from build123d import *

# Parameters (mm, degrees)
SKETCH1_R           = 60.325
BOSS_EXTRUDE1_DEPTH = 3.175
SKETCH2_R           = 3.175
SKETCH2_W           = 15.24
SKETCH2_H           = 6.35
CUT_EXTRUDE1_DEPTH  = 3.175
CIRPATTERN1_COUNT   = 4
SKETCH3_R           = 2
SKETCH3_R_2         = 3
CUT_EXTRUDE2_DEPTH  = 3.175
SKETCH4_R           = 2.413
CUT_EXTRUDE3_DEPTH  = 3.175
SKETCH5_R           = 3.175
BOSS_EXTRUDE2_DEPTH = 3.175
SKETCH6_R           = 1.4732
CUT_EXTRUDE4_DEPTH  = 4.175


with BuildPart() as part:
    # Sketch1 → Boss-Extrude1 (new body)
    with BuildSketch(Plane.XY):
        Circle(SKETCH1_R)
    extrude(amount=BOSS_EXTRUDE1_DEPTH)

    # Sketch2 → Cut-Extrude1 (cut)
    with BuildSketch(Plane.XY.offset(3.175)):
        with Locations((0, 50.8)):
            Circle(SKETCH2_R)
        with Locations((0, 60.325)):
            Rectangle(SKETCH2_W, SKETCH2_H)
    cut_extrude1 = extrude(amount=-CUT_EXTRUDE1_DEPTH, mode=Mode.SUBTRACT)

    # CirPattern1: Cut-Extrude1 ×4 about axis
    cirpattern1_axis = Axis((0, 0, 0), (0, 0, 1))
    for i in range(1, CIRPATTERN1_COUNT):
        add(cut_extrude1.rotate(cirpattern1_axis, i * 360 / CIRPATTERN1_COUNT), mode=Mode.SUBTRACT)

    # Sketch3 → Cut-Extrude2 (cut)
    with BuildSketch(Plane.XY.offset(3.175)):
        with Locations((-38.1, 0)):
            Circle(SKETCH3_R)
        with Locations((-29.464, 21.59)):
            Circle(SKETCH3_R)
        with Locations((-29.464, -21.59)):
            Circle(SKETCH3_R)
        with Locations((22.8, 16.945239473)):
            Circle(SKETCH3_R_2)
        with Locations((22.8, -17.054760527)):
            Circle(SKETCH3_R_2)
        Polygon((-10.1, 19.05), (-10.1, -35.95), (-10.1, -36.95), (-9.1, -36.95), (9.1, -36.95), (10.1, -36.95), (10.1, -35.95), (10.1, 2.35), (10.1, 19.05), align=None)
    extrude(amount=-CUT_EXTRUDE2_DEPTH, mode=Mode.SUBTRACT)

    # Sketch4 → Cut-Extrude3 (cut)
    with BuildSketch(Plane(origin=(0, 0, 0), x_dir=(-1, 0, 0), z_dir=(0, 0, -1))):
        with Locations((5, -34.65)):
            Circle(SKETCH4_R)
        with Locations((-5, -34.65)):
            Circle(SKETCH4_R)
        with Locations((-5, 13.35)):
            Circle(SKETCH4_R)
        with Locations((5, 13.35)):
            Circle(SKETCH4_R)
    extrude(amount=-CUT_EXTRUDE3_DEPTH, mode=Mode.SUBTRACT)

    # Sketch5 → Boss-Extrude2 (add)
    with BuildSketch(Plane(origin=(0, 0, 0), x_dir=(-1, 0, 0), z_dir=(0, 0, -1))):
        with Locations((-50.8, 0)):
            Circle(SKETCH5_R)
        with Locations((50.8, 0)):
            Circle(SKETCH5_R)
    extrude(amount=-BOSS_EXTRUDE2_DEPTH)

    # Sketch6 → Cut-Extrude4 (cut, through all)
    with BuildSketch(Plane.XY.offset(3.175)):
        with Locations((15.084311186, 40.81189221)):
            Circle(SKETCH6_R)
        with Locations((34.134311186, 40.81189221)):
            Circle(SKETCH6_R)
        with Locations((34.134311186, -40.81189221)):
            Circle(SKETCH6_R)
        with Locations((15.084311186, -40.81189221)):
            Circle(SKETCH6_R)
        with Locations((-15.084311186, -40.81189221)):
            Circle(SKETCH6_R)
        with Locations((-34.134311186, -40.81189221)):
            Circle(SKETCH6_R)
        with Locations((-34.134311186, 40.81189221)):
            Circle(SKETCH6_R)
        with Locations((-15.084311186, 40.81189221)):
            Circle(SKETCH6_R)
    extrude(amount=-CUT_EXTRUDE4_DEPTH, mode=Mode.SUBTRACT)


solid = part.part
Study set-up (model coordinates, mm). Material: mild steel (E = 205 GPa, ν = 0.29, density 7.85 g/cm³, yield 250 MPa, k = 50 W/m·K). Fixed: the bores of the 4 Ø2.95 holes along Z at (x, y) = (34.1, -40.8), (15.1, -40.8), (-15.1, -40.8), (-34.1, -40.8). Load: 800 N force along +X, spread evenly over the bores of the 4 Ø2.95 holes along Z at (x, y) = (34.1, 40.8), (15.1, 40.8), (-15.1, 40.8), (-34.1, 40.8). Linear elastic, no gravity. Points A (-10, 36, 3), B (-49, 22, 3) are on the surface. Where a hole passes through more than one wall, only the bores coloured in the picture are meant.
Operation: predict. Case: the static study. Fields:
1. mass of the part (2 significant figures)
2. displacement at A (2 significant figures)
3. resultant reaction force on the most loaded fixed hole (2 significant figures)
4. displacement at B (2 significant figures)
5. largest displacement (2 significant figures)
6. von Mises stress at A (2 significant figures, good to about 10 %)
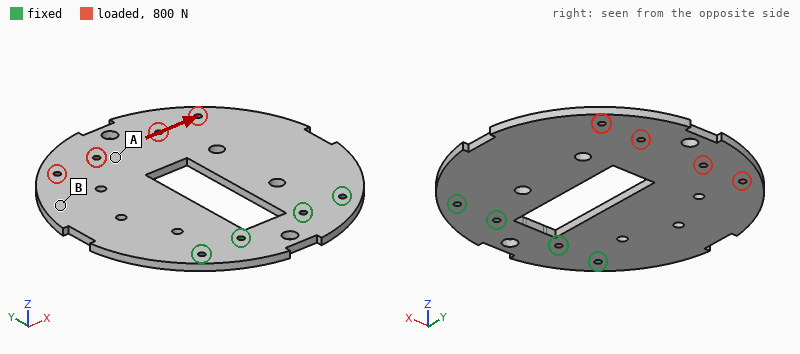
250 g
15 µm
1.1 kN
14 µm
17 µm
11 MPa
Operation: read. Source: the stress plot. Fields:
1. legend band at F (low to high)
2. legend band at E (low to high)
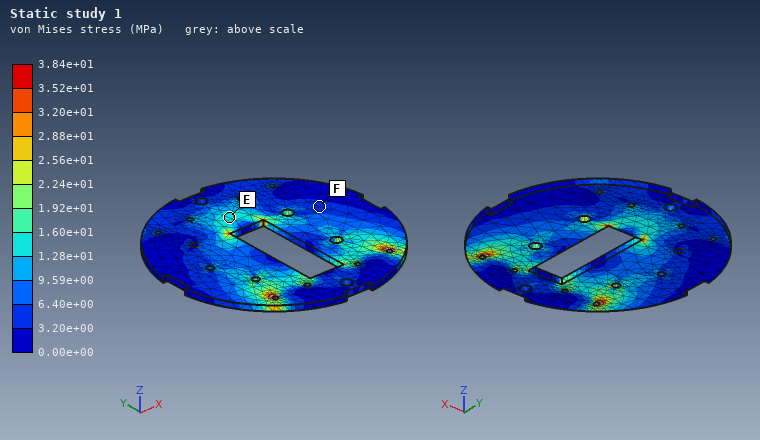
3.20e+00 to 6.40e+00 MPa
1.28e+01 to 1.60e+01 MPa
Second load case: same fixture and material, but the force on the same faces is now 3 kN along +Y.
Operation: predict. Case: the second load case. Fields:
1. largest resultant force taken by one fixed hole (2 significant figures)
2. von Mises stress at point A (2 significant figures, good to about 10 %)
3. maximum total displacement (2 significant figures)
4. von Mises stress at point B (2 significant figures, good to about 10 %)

1000 N
7.6 MPa
6.6 µm
4.1 MPa
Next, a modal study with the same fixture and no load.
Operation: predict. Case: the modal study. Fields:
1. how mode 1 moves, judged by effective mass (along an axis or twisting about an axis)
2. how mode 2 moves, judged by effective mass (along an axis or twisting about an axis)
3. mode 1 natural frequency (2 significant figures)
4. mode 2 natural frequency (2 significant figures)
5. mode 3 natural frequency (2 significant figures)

along Z
twisting about Y
270 Hz
640 Hz
1400 Hz
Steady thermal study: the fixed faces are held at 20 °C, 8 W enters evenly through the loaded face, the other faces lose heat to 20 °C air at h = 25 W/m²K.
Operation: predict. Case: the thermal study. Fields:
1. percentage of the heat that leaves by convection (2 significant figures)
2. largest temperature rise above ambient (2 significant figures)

71 %
25 K
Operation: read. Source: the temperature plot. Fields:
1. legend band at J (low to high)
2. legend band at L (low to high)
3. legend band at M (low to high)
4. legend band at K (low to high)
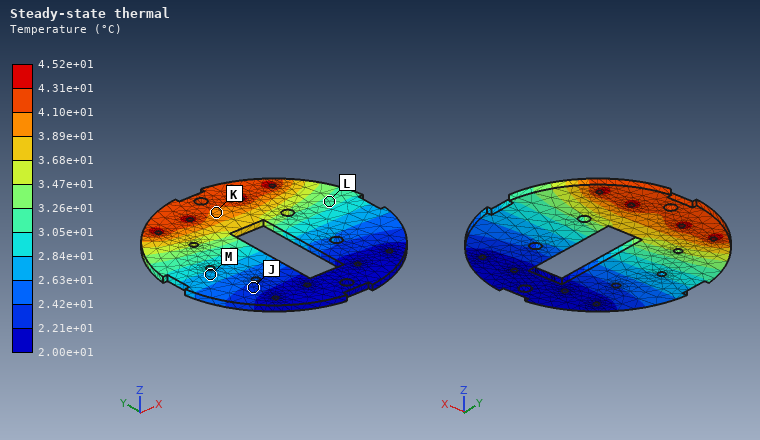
2.21e+01 to 2.42e+01 °C
3.05e+01 to 3.26e+01 °C
2.63e+01 to 2.84e+01 °C
3.89e+01 to 4.10e+01 °C
